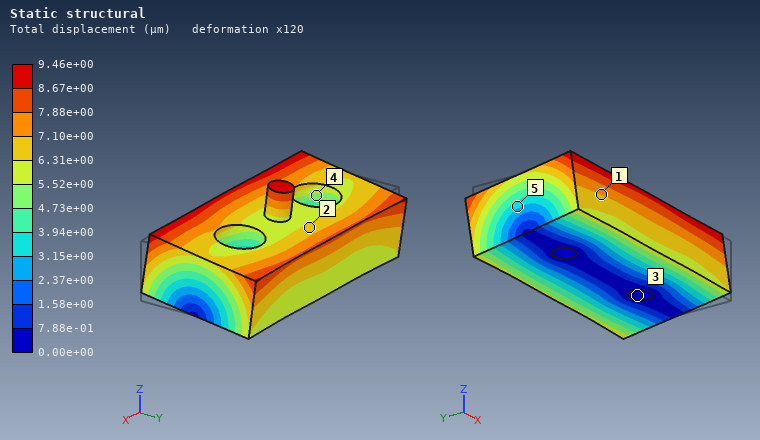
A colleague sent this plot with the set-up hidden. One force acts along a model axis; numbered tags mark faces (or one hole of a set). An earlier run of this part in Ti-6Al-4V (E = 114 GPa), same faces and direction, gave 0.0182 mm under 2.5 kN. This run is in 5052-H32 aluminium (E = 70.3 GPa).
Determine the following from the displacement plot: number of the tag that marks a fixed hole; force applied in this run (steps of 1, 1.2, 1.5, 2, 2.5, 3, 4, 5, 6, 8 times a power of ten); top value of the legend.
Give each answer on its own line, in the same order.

3
800 N
9.46e+00 µm
